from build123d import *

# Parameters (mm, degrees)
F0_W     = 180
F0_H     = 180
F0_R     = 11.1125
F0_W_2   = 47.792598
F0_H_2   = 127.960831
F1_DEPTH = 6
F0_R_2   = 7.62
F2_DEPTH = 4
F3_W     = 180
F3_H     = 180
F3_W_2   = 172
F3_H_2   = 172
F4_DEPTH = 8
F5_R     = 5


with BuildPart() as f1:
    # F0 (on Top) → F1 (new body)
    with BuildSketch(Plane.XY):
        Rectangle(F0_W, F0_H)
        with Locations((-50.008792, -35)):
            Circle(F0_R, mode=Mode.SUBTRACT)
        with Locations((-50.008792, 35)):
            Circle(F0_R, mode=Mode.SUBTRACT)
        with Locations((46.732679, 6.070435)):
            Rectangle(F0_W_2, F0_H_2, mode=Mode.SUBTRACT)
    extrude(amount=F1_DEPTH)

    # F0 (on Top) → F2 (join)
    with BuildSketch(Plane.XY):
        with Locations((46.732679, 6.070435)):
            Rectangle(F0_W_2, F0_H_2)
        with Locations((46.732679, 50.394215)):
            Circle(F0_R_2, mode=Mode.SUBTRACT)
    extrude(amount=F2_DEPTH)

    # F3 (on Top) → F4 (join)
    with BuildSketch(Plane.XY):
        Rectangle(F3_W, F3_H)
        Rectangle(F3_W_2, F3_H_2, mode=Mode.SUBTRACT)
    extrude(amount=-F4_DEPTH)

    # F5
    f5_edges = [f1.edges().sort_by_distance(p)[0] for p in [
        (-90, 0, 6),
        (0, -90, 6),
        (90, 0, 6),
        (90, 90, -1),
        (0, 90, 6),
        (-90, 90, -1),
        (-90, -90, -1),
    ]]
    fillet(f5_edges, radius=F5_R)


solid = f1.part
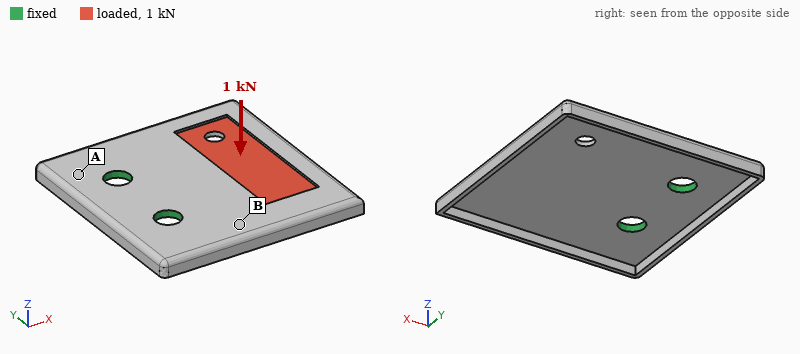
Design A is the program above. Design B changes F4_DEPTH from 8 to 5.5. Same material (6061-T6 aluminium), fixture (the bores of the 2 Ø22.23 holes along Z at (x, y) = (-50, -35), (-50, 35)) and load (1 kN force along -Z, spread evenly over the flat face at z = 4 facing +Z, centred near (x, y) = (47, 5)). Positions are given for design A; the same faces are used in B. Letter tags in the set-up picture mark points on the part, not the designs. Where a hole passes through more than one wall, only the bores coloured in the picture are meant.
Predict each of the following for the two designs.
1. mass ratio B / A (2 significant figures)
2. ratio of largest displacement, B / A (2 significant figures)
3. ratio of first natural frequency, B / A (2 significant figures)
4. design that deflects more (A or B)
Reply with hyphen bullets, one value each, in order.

- 0.96
- 1.2
- 0.97
- B
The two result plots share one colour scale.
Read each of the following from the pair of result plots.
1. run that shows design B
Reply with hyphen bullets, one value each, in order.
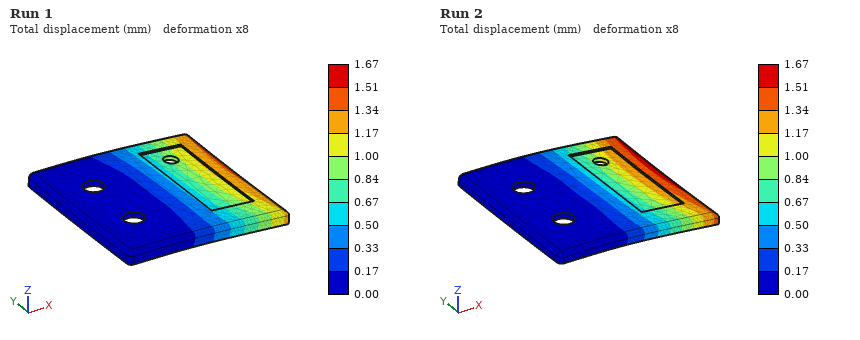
- Run 2
